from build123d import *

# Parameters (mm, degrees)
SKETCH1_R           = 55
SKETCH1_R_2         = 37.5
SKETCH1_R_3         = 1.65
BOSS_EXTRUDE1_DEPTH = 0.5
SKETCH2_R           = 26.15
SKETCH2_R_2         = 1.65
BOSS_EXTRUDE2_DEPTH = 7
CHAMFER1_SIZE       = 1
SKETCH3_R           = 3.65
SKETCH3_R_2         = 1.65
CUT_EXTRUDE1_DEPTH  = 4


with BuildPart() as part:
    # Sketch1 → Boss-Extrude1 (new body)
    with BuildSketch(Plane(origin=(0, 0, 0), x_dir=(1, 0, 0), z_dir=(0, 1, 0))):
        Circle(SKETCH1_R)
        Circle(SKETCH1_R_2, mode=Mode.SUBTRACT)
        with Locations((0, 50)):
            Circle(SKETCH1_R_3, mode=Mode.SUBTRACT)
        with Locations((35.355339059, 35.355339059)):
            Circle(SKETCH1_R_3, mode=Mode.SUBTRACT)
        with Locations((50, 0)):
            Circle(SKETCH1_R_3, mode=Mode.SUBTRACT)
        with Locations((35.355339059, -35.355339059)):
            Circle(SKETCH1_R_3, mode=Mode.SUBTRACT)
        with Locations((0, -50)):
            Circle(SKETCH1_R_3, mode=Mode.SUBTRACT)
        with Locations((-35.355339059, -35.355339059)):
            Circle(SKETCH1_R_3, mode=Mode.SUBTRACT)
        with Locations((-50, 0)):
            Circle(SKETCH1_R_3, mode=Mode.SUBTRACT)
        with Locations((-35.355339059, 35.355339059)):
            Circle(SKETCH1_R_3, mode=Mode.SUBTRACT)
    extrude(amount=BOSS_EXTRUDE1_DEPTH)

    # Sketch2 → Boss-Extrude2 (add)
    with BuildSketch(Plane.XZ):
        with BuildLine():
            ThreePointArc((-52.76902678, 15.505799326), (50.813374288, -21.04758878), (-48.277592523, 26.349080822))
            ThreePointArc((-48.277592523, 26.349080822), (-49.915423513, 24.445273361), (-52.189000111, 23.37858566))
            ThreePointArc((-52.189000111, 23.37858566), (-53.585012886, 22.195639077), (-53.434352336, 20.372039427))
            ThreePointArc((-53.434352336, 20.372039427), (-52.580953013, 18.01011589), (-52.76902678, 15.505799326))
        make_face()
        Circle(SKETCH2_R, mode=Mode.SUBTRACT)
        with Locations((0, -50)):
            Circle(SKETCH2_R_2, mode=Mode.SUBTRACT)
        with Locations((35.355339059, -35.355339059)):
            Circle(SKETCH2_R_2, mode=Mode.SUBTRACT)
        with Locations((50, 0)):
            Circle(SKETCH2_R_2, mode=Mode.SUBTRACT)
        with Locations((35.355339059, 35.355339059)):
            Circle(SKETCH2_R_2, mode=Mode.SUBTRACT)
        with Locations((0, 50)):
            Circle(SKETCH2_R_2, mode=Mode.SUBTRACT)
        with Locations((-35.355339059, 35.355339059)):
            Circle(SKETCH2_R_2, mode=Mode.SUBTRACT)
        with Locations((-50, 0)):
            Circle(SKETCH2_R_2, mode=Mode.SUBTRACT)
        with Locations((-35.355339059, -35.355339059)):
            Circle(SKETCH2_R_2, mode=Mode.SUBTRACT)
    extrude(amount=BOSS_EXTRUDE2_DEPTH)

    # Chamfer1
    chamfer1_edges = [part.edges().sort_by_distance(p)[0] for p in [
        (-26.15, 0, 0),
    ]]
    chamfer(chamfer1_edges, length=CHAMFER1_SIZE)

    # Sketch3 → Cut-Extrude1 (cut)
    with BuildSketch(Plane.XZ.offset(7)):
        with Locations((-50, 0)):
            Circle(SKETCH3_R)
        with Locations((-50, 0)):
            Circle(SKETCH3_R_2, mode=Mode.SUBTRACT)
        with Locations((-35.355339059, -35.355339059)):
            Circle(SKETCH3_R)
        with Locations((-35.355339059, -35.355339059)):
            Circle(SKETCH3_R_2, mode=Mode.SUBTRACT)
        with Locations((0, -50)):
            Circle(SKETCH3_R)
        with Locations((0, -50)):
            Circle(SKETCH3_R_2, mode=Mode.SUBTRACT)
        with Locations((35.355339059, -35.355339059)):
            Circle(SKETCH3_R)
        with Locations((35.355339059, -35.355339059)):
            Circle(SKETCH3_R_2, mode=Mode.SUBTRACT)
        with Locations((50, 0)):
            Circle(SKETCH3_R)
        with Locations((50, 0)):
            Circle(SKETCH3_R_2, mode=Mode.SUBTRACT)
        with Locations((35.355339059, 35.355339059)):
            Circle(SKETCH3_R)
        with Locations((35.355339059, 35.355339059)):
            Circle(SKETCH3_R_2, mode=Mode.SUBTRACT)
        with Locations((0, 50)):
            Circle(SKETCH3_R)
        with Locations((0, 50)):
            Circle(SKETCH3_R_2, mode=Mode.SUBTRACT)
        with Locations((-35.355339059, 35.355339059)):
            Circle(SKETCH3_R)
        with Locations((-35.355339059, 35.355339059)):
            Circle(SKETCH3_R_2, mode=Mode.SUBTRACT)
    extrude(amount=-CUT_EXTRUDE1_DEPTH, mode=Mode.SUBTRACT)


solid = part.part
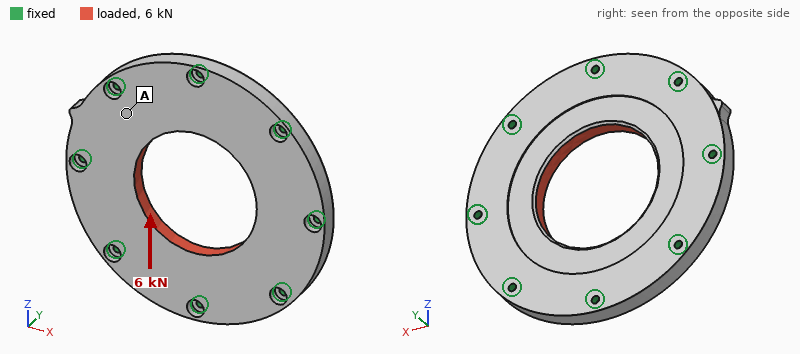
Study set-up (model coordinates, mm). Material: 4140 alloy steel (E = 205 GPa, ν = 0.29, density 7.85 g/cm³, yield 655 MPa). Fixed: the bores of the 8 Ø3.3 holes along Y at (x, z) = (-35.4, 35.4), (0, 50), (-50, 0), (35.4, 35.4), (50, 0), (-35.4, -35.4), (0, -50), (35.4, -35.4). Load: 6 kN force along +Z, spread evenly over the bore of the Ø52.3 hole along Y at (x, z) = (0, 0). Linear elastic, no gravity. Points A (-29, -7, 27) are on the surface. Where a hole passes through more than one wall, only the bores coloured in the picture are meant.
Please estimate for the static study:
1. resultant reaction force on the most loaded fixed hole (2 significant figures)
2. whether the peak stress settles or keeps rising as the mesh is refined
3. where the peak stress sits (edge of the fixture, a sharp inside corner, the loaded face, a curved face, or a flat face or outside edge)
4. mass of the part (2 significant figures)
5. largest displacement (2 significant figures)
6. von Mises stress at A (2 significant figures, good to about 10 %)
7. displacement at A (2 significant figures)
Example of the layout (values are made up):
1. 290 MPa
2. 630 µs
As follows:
1. 950 N
2. keeps rising
3. edge of the fixture
4. 410 g
5. 3.0 µm
6. 5.8 MPa
7. 1.2 µm
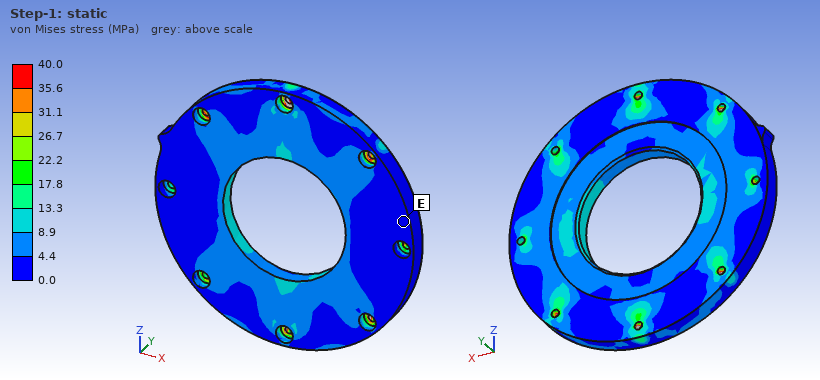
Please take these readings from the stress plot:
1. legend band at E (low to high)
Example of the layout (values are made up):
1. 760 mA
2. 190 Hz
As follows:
1. 0.0 to 4.4 MPa
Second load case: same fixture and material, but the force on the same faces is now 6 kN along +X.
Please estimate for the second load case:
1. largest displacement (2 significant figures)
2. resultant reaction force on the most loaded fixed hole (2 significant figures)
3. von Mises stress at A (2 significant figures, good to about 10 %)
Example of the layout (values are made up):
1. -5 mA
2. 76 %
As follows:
1. 3.0 µm
2. 950 N
3. 5.8 MPa
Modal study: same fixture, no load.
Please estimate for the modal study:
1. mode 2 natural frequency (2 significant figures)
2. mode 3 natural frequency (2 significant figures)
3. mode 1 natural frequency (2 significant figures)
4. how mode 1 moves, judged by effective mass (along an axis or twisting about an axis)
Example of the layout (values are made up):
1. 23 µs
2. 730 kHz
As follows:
1. 8900 Hz
2. 8900 Hz
3. 6400 Hz
4. along Y
